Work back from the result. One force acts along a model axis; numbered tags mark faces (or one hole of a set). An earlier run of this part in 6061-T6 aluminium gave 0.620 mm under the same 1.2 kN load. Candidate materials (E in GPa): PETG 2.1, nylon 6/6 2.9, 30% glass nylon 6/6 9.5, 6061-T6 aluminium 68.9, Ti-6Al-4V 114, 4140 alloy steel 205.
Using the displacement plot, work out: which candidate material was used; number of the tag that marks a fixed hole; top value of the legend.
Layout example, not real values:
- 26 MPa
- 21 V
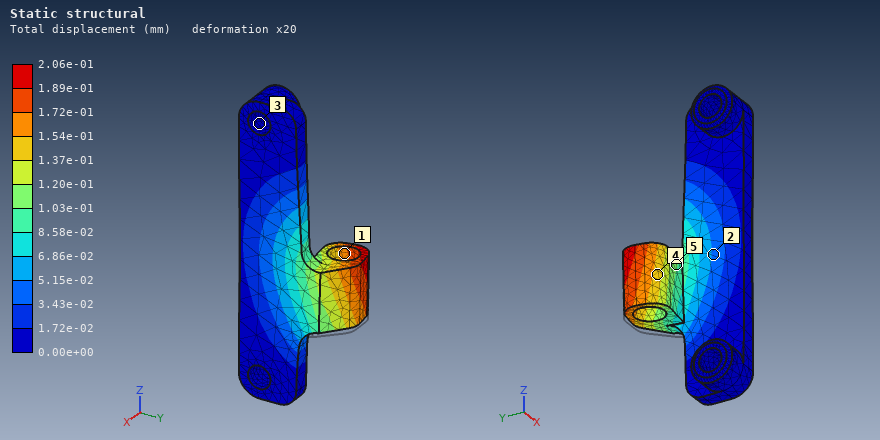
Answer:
- 4140 alloy steel
- 3
- 2.06e-01 mm
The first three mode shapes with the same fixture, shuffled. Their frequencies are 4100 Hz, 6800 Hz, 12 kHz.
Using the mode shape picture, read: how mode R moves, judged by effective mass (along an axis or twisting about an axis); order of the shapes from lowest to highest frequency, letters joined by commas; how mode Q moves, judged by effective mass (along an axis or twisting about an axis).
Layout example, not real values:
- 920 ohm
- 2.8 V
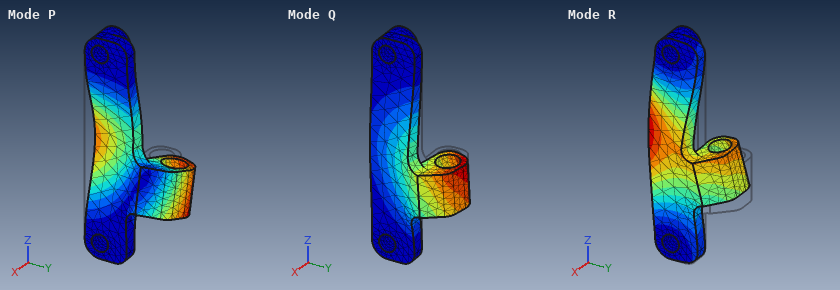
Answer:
- along Y
- Q, P, R
- along X
